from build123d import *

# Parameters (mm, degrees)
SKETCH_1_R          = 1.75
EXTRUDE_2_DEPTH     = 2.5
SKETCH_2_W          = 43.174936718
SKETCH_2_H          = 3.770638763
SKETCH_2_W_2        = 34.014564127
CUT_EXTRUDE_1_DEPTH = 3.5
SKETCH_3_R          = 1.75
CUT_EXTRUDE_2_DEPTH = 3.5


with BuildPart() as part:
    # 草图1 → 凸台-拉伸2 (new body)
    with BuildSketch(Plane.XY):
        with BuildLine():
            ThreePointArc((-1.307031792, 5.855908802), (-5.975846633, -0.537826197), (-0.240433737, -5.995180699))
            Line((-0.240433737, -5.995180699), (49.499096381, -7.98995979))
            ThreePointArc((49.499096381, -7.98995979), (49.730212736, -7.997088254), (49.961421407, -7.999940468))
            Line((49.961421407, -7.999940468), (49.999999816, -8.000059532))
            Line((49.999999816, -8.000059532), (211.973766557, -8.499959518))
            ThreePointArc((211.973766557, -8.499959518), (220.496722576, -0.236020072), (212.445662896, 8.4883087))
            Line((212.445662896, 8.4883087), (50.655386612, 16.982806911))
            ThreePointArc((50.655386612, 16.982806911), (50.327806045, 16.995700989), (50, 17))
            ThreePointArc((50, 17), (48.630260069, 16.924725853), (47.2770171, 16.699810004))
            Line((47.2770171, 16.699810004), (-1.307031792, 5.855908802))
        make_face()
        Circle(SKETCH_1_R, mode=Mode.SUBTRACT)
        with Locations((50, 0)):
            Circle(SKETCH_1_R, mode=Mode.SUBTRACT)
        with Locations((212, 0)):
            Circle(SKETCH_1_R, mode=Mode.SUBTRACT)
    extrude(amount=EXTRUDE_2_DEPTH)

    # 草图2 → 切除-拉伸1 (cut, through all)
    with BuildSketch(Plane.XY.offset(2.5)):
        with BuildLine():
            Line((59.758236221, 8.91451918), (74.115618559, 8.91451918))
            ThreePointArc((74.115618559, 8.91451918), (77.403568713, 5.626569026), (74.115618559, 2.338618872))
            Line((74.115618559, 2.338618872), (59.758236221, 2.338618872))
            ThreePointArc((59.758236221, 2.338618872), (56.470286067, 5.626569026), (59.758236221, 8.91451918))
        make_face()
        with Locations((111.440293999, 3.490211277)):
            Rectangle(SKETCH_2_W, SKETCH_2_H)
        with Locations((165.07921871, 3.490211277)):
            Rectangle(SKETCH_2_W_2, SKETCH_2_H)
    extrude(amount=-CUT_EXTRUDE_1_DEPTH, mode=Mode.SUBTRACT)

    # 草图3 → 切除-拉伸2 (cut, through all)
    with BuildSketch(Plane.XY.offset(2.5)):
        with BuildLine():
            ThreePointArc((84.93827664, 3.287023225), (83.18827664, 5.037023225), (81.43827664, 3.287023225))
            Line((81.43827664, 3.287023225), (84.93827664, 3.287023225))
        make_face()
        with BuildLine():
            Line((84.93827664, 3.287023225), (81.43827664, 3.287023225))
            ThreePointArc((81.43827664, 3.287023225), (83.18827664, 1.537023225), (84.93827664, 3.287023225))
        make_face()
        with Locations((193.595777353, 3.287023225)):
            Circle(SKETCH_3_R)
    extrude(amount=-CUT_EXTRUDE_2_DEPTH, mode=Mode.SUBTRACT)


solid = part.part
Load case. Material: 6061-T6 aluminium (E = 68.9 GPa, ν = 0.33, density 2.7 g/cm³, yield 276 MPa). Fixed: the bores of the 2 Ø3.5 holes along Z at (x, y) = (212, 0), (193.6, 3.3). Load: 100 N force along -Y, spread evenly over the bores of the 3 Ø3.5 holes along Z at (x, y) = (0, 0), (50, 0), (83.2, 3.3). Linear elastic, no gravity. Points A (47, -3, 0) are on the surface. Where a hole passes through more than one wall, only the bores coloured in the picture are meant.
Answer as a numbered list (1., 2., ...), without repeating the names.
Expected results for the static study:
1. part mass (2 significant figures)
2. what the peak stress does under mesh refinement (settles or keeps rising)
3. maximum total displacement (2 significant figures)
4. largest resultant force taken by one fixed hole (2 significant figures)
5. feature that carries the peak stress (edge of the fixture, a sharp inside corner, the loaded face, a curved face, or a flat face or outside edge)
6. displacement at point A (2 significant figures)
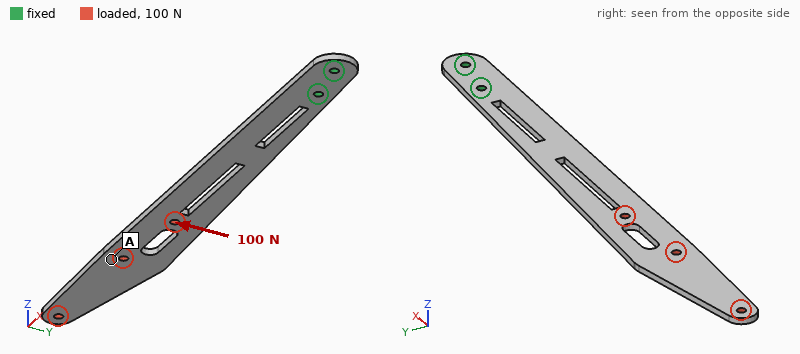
1. 27 g
2. keeps rising
3. 2.0 mm
4. 800 N
5. edge of the fixture
6. 1.3 mm
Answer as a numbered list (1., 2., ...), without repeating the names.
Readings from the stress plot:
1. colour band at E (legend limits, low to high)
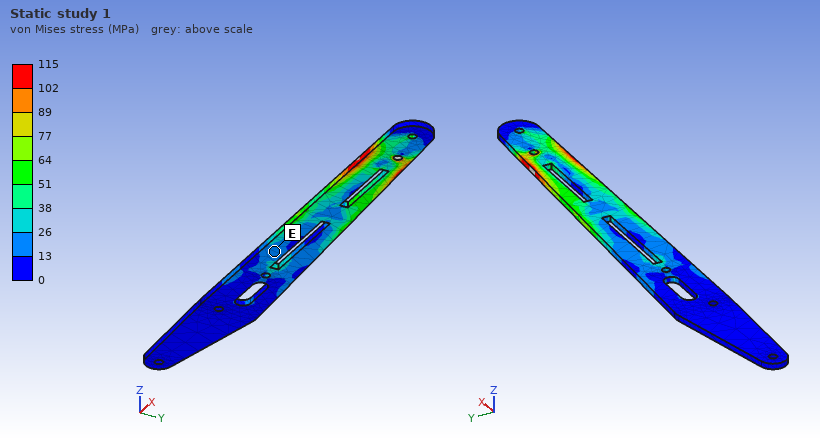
1. 13 to 26 MPa
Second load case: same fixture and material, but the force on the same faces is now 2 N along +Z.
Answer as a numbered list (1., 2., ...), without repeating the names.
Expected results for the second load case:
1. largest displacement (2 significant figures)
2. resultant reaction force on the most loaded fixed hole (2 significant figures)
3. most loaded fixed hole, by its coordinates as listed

1. 2.2 mm
2. 5.9 N
3. (193.6, 3.3)
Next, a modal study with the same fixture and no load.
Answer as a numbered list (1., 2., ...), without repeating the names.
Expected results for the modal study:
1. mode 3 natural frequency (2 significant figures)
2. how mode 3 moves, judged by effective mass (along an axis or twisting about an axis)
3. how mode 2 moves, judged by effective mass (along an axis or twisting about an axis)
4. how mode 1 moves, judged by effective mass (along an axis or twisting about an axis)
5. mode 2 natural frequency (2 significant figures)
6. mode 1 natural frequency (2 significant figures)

1. 370 Hz
2. along Y
3. along Z
4. along Z
5. 340 Hz
6. 51 Hz
